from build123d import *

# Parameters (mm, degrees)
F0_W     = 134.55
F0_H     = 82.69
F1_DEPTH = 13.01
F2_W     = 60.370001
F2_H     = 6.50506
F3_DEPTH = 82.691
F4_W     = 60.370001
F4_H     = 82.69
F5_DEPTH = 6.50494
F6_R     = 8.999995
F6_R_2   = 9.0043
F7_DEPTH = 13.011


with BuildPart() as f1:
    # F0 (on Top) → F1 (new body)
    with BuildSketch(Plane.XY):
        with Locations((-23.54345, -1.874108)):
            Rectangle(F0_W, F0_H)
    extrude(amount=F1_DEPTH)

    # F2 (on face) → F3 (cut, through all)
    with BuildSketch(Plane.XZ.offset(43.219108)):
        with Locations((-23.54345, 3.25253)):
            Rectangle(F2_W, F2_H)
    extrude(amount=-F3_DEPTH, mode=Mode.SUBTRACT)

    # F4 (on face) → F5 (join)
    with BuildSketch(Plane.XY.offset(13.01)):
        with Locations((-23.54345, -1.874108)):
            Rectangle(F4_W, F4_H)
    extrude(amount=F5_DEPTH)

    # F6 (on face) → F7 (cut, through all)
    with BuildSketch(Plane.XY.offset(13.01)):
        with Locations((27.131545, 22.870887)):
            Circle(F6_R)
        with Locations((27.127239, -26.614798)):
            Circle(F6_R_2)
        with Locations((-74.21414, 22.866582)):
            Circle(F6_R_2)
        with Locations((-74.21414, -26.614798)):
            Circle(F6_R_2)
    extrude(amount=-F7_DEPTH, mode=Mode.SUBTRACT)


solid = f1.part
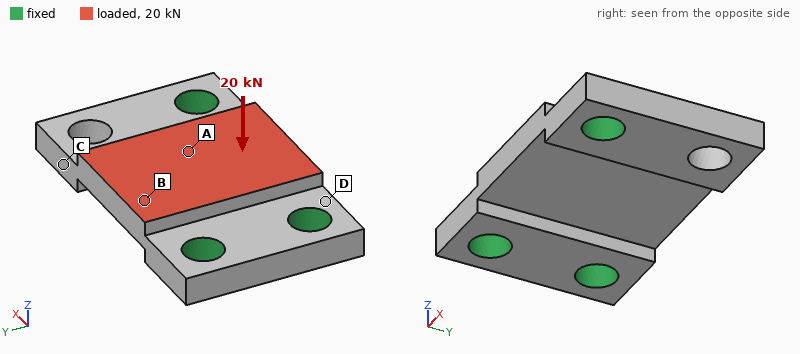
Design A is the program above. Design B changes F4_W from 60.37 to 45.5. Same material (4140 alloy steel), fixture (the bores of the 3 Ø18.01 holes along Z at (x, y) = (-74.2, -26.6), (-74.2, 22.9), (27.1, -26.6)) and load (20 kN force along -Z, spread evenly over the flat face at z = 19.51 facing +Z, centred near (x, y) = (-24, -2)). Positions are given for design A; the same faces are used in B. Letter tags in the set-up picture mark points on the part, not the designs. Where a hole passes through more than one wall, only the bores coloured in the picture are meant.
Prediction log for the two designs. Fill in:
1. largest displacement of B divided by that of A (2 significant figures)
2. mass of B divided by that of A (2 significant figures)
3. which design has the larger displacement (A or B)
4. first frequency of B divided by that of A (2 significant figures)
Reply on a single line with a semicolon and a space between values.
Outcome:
1.3; 0.94; B; 0.96
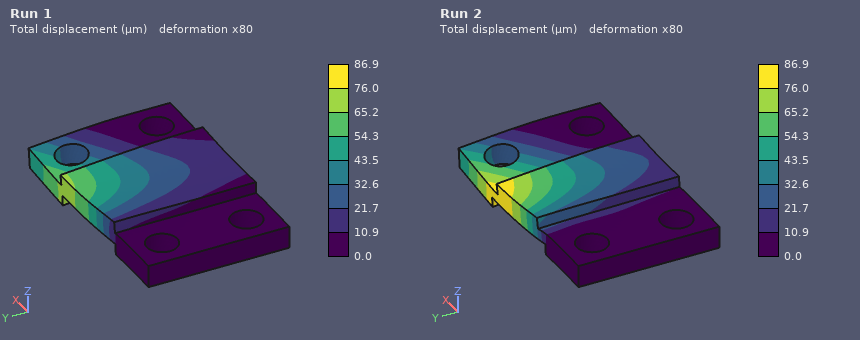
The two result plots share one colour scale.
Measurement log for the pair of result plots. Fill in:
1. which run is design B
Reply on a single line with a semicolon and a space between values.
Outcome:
Run 2
